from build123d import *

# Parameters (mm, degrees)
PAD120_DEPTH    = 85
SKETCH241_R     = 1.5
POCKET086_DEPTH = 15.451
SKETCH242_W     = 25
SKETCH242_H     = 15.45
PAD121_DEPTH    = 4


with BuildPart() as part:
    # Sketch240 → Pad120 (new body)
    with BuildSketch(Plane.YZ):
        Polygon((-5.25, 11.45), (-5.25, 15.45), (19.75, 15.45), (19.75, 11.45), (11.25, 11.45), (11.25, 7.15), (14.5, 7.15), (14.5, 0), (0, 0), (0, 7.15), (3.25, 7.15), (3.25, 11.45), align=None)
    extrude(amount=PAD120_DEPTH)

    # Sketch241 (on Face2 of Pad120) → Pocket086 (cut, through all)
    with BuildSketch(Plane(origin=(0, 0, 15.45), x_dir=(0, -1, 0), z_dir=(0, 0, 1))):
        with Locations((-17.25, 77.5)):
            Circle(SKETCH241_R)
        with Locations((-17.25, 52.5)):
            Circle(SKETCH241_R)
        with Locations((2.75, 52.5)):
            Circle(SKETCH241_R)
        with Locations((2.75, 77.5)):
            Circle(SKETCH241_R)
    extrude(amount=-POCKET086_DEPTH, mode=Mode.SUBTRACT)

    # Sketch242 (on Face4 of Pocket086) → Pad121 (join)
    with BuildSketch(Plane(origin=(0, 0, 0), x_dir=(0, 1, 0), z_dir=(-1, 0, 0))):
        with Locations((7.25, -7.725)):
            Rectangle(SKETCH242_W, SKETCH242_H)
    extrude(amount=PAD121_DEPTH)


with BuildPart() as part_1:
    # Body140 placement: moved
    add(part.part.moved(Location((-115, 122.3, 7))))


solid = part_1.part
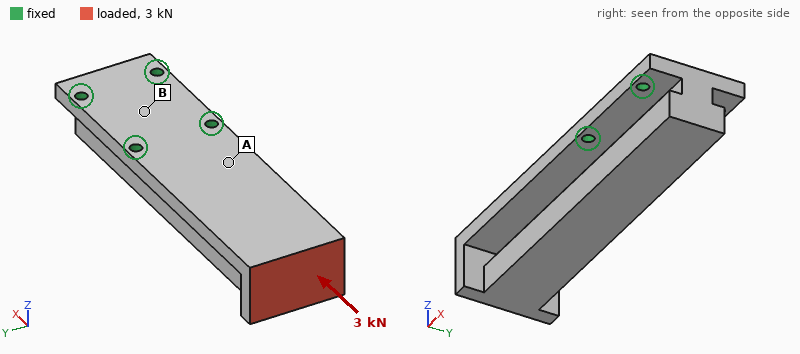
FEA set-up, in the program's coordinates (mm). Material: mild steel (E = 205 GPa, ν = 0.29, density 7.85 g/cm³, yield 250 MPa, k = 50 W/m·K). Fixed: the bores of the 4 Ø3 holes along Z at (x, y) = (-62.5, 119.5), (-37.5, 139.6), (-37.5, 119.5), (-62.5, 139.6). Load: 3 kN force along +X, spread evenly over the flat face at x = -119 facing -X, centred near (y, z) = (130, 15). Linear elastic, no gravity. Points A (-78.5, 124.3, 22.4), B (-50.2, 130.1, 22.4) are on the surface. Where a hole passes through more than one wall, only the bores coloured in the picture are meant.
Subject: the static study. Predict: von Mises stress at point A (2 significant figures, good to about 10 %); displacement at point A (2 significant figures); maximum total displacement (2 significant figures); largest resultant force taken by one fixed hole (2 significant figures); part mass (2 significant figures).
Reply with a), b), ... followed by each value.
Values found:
a) 11 MPa
b) 5.0 µm
c) 22 µm
d) 1.1 kN
e) 170 g
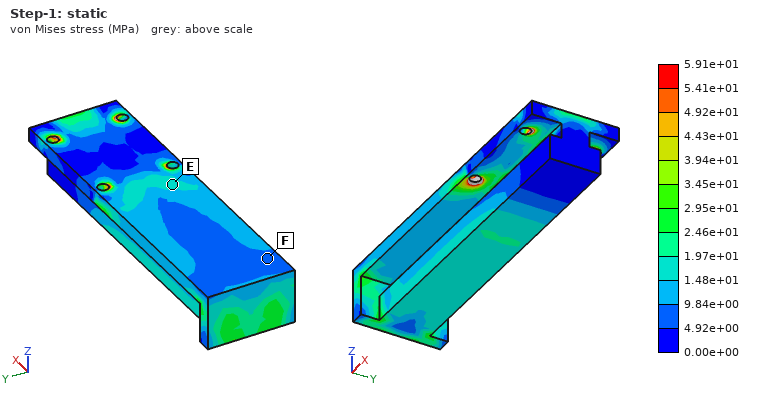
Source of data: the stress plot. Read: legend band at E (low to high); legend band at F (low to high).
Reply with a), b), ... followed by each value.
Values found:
a) 1.48e+01 to 1.97e+01 MPa
b) 4.92e+00 to 9.84e+00 MPa
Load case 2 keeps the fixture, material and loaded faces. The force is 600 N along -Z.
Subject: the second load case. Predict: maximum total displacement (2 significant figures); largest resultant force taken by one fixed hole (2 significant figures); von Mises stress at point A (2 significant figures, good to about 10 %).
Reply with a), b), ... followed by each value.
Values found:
a) 69 µm
b) 1.1 kN
c) 32 MPa
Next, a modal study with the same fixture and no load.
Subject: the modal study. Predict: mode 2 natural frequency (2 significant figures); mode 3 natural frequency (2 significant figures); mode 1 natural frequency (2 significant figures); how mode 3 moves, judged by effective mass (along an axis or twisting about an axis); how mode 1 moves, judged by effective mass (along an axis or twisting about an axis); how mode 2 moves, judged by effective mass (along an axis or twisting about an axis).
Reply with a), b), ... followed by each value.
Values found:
a) 3800 Hz
b) 6700 Hz
c) 2400 Hz
d) twisting about X
e) along Z
f) along Y
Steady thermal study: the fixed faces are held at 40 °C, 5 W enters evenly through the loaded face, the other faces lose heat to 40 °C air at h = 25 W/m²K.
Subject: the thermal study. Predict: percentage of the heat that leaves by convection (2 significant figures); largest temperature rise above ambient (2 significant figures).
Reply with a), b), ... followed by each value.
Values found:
a) 33 %
b) 22 K
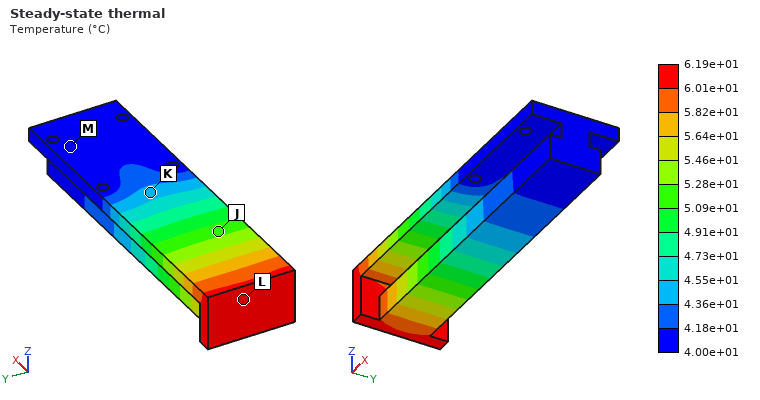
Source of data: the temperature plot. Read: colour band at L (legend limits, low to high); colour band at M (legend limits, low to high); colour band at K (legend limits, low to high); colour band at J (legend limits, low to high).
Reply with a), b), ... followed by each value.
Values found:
a) 6.01e+01 to 6.19e+01 °C
b) 4.00e+01 to 4.18e+01 °C
c) 4.36e+01 to 4.55e+01 °C
d) 5.09e+01 to 5.28e+01 °C
